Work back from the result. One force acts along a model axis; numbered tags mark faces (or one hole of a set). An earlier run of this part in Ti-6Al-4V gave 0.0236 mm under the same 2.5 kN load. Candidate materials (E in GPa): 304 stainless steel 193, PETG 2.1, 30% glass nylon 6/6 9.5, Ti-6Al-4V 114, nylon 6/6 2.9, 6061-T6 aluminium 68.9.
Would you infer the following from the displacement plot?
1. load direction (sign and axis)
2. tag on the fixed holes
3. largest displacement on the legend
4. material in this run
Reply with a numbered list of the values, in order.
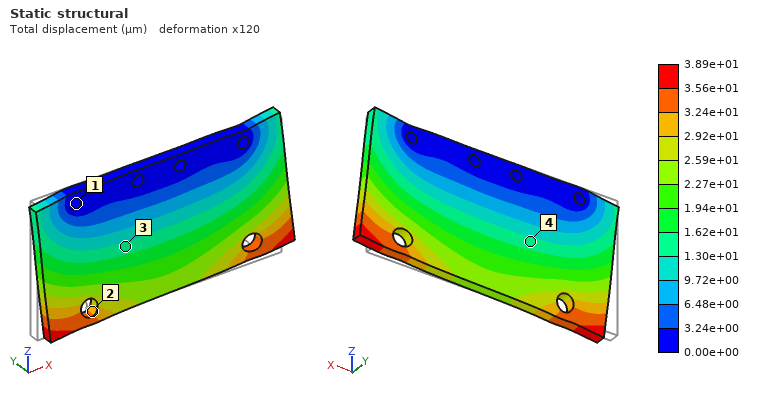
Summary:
1. +X
2. 1
3. 3.89e+01 µm
4. 6061-T6 aluminium
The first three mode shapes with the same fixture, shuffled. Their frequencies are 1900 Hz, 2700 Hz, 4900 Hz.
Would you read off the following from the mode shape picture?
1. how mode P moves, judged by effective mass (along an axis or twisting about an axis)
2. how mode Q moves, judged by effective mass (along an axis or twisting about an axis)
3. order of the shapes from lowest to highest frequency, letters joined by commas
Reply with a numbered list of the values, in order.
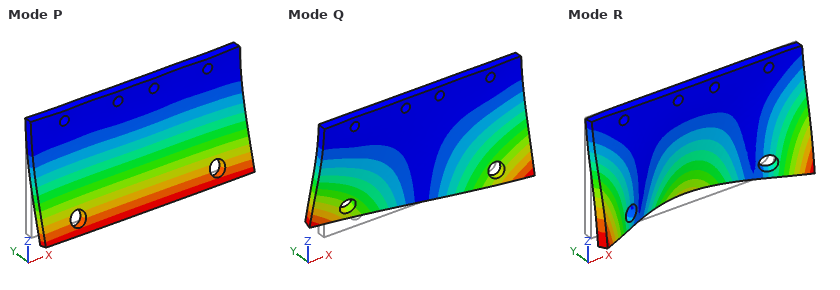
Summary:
1. along Y
2. twisting about Z
3. P, Q, R
